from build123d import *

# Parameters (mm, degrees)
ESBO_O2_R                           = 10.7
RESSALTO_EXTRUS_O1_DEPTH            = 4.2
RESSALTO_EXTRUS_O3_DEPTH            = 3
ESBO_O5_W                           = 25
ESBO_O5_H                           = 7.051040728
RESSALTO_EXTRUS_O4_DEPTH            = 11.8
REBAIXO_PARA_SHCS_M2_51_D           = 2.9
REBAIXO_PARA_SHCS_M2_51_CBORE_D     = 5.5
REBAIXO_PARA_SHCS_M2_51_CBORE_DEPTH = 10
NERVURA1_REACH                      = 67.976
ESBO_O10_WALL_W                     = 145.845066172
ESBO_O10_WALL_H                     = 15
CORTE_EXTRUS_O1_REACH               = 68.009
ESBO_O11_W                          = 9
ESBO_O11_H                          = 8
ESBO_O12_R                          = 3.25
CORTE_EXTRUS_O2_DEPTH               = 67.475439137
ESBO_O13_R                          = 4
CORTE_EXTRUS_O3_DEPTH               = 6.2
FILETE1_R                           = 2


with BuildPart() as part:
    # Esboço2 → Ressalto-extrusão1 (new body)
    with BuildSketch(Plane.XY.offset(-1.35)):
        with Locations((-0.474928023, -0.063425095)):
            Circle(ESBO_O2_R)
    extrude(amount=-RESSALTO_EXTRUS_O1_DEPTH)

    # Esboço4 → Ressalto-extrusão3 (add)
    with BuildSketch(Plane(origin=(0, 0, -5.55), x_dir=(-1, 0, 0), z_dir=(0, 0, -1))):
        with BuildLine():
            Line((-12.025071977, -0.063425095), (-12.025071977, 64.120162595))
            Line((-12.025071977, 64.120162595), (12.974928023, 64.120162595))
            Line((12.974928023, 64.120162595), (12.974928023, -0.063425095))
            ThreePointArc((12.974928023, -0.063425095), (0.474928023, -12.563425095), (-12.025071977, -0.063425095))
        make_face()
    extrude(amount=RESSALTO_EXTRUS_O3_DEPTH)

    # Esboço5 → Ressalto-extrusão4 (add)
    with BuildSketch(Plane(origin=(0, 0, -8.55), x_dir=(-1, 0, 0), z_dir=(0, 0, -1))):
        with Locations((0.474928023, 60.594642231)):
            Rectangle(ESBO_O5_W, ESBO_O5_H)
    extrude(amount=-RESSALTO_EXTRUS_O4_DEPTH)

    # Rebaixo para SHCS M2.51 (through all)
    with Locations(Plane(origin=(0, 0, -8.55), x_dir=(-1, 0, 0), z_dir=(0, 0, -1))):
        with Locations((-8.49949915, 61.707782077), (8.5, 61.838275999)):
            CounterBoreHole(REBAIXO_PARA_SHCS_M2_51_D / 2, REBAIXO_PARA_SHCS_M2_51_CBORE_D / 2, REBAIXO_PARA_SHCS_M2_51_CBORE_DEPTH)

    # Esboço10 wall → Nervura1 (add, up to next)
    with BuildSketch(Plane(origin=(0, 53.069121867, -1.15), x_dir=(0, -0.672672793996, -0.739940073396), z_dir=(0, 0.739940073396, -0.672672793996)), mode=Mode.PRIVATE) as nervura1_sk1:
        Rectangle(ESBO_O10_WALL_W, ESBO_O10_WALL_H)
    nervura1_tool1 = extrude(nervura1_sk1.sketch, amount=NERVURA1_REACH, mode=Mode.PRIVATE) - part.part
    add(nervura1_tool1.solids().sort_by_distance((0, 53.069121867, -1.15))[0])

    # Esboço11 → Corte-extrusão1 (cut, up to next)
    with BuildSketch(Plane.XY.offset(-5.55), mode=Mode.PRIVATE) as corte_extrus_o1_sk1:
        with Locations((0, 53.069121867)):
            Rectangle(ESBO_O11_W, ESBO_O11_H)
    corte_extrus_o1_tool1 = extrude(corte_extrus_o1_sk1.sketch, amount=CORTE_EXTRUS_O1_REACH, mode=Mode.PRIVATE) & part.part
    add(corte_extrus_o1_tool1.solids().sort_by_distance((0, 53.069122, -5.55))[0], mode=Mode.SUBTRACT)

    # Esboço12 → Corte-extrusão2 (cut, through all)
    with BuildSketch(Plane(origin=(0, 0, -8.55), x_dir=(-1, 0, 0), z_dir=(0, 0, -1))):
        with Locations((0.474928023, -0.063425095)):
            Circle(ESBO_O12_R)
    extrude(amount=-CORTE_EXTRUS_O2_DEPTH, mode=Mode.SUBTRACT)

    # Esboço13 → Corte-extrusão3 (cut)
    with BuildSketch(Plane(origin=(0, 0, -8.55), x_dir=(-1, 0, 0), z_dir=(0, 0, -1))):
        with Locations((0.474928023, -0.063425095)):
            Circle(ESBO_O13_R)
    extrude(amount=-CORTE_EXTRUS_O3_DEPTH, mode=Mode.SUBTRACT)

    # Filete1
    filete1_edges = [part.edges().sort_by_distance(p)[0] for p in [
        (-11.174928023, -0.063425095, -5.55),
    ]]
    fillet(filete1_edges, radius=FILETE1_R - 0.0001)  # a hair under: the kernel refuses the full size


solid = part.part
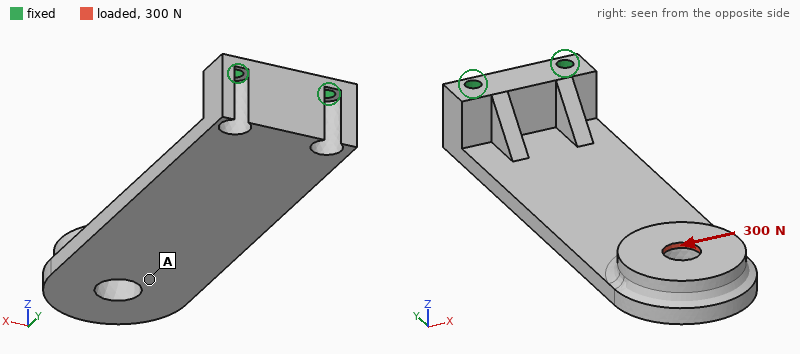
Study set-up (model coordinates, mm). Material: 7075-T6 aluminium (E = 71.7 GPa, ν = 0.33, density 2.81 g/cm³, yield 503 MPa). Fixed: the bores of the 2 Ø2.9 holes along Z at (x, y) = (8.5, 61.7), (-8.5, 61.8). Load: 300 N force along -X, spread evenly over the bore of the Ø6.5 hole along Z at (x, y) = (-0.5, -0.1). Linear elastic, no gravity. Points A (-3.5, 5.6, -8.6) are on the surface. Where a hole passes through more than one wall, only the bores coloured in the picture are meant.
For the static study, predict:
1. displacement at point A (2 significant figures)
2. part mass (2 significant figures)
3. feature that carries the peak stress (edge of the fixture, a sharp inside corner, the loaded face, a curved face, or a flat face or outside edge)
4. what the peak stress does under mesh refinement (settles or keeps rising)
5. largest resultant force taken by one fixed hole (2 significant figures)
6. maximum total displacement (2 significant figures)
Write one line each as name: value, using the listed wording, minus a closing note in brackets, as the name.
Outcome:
displacement at point A: 0.26 mm
part mass: 23 g
feature that carries the peak stress: edge of the fixture
what the peak stress does under mesh refinement: keeps rising
largest resultant force taken by one fixed hole: 1.0 kN
maximum total displacement: 0.46 mm
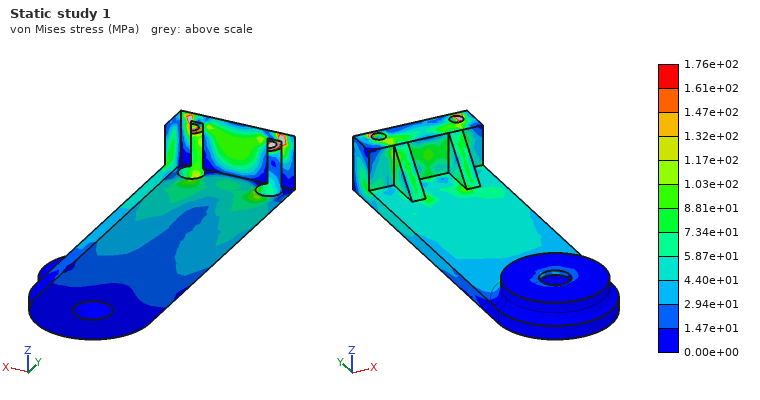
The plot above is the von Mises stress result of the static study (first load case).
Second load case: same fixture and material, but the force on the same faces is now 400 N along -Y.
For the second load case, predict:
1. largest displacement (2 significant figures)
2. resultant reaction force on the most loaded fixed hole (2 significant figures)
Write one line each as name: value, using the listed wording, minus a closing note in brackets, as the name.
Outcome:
largest displacement: 0.81 mm
resultant reaction force on the most loaded fixed hole: 220 N
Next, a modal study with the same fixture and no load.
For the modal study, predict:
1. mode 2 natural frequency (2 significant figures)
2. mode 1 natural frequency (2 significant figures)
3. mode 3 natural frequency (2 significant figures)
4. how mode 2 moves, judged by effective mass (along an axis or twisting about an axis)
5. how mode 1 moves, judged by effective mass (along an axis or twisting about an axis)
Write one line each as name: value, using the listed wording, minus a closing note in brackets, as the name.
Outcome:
mode 2 natural frequency: 1500 Hz
mode 1 natural frequency: 410 Hz
mode 3 natural frequency: 2400 Hz
how mode 2 moves, judged by effective mass: along X
how mode 1 moves, judged by effective mass: along Z
